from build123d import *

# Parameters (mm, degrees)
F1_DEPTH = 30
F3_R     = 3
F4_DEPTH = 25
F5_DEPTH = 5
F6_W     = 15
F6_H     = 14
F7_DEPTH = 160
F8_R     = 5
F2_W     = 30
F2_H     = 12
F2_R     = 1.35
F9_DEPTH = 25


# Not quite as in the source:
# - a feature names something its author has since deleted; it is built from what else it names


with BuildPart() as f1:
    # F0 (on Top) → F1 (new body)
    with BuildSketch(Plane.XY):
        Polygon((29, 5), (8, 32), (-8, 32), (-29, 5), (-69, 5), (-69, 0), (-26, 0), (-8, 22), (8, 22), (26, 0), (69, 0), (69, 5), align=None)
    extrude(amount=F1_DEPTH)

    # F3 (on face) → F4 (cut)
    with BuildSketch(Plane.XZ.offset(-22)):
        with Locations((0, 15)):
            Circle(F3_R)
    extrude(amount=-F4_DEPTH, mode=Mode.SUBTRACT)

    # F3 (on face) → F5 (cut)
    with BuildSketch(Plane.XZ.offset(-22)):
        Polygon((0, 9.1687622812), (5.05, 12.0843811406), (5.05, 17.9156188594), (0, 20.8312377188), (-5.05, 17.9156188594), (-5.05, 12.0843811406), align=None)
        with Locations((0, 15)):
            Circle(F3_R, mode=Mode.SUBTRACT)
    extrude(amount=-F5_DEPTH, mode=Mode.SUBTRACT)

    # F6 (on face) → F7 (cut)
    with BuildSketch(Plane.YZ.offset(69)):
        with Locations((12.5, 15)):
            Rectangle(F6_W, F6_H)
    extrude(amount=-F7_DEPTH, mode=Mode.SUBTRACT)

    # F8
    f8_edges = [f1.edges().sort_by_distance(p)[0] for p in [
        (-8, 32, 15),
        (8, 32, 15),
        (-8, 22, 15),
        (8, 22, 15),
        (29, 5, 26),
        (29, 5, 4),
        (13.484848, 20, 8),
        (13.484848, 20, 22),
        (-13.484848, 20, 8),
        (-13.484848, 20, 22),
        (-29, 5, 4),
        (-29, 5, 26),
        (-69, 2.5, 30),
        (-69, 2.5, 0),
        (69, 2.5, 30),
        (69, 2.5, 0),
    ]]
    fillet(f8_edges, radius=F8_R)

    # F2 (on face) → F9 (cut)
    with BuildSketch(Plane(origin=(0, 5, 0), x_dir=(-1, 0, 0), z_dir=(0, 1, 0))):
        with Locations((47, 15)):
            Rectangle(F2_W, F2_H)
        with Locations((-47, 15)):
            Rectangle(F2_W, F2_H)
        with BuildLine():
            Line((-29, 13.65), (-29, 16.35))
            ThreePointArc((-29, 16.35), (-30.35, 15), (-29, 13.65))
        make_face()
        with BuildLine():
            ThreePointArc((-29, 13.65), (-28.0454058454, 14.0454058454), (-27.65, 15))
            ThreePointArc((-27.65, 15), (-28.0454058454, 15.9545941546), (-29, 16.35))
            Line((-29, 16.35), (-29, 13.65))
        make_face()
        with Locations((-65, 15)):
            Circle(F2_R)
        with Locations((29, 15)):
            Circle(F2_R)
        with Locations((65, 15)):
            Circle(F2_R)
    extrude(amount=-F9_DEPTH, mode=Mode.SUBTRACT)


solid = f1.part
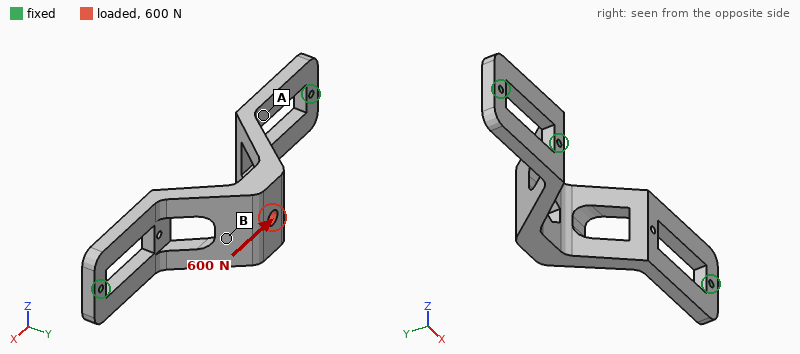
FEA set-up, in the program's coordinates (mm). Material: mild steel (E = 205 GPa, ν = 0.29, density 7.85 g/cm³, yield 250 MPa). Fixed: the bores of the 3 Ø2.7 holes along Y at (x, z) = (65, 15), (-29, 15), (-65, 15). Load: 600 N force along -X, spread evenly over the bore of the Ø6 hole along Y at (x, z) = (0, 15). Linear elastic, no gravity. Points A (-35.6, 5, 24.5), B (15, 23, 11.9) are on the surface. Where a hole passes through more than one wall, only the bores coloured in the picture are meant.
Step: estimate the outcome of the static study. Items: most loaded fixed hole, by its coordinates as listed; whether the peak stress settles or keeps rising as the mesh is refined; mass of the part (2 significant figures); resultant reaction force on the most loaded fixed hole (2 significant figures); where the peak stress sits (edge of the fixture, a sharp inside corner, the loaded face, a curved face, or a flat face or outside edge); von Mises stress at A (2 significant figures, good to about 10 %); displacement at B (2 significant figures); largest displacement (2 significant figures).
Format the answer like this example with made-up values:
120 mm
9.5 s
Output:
(65, 15)
keeps rising
160 g
400 N
edge of the fixture
10 MPa
34 µm
37 µm
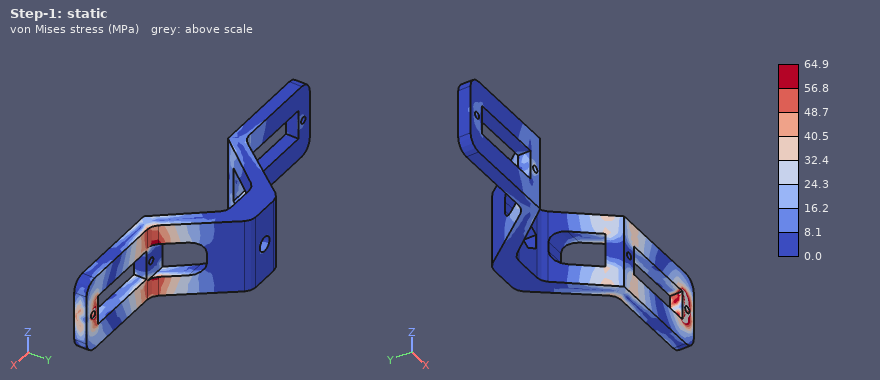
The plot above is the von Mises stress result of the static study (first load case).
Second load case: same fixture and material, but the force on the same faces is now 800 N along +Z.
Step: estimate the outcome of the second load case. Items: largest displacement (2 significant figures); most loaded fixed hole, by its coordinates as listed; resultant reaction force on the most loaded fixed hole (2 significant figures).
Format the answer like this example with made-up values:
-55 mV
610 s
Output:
0.10 mm
(-29, 15)
990 N
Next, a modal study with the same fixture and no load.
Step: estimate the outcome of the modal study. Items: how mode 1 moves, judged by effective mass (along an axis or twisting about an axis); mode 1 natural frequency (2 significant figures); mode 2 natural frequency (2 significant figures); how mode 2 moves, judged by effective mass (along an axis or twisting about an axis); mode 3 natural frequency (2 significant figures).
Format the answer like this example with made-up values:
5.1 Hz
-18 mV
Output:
along Y
1800 Hz
1900 Hz
along Z
3400 Hz
